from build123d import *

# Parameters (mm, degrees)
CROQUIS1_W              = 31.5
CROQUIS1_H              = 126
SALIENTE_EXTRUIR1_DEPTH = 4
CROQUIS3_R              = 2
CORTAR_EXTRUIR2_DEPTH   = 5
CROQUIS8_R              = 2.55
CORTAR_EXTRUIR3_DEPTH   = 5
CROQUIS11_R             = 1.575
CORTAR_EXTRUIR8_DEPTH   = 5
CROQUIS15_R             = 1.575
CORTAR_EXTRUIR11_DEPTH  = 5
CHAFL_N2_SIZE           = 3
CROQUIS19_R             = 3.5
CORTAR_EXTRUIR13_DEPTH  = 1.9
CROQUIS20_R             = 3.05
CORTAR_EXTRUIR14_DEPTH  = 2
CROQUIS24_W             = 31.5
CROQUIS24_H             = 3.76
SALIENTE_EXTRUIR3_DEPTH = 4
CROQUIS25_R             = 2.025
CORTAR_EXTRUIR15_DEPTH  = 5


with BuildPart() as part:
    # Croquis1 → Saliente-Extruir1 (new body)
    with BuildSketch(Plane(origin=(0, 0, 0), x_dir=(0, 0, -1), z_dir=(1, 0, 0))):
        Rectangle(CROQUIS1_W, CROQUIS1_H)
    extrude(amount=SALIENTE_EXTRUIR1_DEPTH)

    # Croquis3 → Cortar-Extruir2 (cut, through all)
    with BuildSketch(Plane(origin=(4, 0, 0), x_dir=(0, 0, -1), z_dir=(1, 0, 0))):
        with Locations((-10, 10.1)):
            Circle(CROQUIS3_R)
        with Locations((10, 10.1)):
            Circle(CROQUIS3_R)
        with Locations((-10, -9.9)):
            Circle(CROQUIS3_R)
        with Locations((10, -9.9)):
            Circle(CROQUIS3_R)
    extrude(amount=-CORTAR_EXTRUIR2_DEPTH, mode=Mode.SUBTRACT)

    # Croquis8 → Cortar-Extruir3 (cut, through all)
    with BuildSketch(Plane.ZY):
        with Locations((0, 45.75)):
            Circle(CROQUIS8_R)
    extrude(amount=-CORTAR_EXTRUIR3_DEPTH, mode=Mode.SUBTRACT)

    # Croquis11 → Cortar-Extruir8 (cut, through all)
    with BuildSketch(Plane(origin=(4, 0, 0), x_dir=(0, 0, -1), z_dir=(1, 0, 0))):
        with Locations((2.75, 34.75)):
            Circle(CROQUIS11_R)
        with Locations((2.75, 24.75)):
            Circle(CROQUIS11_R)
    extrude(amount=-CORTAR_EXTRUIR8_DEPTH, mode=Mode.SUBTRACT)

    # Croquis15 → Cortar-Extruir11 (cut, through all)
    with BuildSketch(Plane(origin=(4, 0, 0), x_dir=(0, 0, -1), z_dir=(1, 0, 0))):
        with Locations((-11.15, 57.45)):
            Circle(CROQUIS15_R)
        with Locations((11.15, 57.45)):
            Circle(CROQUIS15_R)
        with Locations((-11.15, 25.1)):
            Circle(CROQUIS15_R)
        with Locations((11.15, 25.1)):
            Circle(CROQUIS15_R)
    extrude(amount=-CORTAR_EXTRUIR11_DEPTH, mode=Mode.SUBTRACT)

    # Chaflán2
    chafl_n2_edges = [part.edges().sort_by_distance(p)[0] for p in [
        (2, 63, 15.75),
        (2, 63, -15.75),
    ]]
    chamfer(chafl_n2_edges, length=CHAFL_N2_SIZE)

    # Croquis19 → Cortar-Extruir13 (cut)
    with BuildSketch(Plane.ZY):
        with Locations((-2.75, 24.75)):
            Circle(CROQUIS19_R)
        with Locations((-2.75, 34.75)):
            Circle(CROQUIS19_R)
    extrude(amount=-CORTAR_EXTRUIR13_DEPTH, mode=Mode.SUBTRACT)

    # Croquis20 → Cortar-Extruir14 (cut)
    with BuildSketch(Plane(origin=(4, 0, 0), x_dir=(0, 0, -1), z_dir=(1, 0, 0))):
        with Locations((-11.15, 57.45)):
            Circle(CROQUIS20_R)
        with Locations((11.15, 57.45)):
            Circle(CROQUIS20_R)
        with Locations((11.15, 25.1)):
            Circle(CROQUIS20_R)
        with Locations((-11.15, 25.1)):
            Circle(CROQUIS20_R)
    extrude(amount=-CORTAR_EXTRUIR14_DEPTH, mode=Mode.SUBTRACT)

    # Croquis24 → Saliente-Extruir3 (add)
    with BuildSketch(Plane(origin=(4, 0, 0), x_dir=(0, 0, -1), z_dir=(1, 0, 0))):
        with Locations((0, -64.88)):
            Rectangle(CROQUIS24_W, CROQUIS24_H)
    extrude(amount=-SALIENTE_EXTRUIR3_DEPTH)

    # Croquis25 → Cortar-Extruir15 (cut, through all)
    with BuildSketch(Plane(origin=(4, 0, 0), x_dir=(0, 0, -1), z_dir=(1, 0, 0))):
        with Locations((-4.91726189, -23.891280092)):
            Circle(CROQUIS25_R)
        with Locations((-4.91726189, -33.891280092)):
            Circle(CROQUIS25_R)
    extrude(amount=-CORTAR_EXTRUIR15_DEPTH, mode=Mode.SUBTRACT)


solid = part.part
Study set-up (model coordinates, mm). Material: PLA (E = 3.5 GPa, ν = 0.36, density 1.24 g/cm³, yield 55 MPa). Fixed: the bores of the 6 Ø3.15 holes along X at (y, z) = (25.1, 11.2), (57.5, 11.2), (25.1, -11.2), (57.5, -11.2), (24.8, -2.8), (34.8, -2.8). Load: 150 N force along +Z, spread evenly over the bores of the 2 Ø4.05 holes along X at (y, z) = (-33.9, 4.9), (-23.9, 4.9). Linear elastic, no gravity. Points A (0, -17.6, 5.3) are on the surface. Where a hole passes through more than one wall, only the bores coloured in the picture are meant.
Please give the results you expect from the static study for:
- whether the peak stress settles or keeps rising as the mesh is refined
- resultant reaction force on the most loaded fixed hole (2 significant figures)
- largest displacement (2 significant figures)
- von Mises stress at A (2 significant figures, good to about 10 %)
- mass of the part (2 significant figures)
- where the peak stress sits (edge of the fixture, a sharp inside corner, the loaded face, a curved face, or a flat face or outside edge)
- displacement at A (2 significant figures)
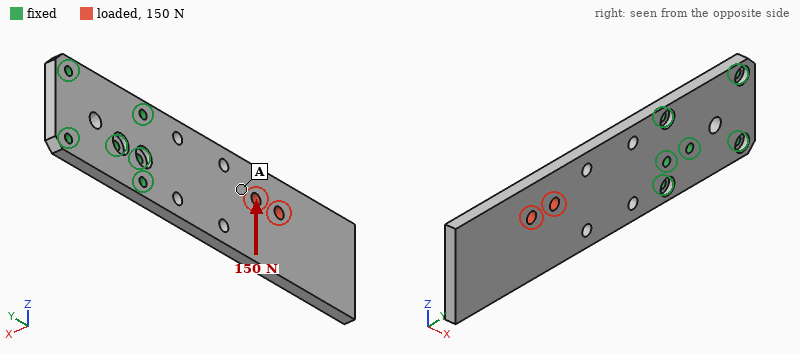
keeps rising
300 N
0.69 mm
2.9 MPa
19 g
edge of the fixture
0.28 mm
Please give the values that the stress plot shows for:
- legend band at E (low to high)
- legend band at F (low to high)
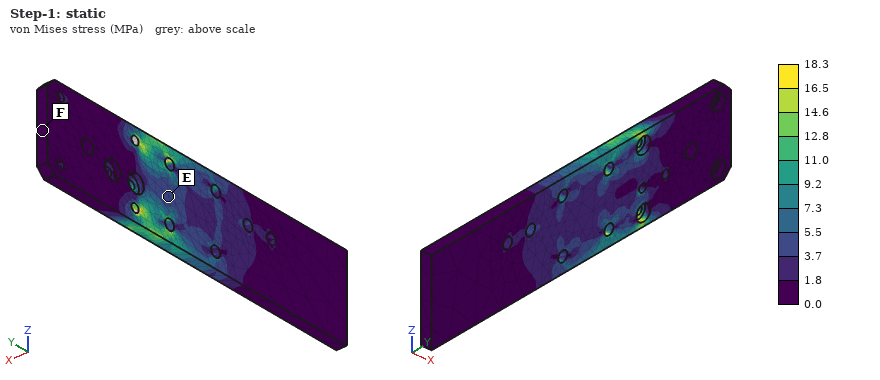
3.7 to 5.5 MPa
0.0 to 1.8 MPa
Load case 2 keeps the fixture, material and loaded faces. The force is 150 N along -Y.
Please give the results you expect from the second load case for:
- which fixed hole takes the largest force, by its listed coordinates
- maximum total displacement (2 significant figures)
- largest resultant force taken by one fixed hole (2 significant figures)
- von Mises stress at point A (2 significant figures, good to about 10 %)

(25.1, 11.2)
0.11 mm
74 N
1.9 MPa
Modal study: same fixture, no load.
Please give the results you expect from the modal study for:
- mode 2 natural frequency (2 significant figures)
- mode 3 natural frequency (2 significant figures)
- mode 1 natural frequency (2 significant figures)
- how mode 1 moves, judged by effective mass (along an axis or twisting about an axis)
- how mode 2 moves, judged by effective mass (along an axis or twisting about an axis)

690 Hz
760 Hz
120 Hz
along X
twisting about Y
